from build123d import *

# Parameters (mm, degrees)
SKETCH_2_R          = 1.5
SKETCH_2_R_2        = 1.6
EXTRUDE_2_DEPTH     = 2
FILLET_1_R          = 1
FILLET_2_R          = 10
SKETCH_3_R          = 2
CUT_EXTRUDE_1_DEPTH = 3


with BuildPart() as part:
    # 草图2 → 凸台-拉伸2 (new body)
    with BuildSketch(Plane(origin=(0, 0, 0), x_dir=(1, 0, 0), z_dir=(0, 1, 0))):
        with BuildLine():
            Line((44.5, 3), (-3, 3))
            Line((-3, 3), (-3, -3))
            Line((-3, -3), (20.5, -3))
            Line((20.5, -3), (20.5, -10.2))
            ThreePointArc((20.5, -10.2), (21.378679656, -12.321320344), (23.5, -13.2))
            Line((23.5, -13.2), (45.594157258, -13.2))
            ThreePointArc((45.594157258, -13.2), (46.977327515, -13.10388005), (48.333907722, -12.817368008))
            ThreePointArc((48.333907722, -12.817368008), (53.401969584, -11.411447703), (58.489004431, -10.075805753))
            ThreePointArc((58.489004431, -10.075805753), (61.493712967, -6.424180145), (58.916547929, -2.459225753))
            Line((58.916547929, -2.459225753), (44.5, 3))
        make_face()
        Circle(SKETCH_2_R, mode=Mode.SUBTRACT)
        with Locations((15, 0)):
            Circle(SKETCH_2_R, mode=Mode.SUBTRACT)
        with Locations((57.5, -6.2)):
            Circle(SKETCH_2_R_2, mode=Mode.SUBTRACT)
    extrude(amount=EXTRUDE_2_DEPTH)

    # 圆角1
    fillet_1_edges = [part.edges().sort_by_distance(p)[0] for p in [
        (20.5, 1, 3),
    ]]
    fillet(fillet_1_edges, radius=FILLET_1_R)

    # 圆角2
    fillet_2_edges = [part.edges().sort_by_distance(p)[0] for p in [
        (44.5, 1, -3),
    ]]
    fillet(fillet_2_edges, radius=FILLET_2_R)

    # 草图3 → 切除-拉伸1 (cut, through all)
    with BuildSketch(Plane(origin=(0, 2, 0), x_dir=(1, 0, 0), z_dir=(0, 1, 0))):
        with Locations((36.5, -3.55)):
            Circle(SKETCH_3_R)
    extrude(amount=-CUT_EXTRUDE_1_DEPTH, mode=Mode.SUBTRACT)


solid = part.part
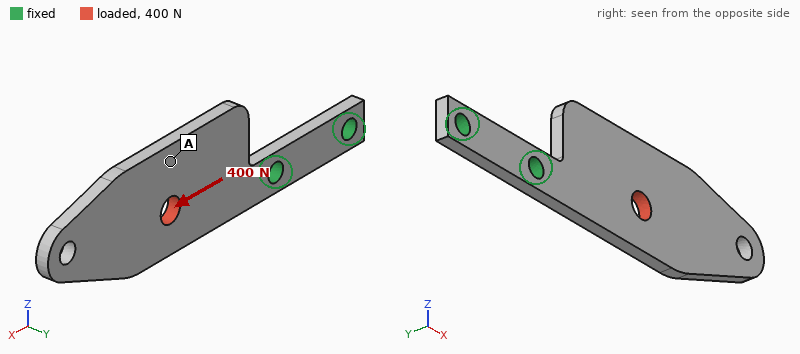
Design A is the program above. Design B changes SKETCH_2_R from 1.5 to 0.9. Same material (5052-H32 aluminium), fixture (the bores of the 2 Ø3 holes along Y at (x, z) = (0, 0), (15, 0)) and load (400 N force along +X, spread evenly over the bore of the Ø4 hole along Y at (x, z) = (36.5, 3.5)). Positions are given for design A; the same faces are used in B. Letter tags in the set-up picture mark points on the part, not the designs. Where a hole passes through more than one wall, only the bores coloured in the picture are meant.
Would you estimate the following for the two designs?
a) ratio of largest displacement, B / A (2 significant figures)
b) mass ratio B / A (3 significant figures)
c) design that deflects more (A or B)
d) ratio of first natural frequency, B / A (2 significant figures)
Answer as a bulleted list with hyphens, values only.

- 1.2
- 1.01
- B
- 0.95
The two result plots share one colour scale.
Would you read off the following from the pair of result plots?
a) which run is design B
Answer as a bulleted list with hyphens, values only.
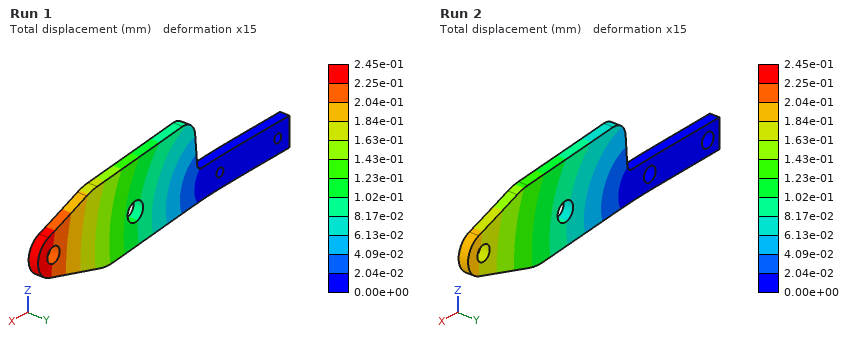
- Run 1
